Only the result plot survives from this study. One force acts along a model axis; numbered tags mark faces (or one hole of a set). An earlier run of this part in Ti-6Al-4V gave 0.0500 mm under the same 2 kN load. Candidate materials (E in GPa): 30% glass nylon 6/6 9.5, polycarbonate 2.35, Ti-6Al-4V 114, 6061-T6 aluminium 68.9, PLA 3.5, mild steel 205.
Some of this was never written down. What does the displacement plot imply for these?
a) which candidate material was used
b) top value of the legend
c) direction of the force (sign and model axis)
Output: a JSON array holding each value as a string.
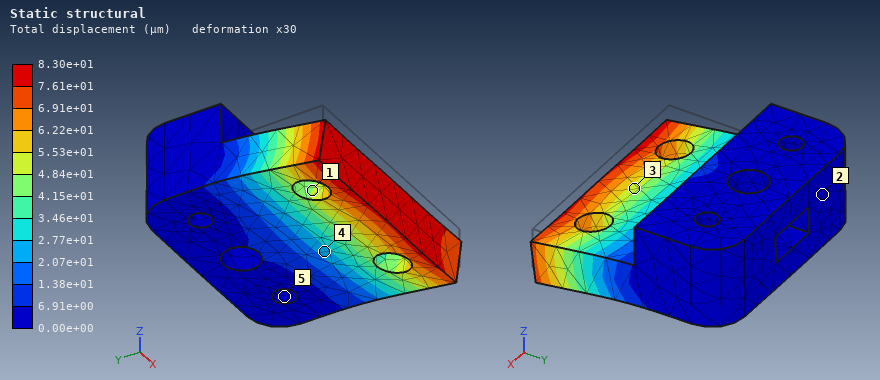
["6061-T6 aluminium", "8.30e+01 µm", "-Z"]
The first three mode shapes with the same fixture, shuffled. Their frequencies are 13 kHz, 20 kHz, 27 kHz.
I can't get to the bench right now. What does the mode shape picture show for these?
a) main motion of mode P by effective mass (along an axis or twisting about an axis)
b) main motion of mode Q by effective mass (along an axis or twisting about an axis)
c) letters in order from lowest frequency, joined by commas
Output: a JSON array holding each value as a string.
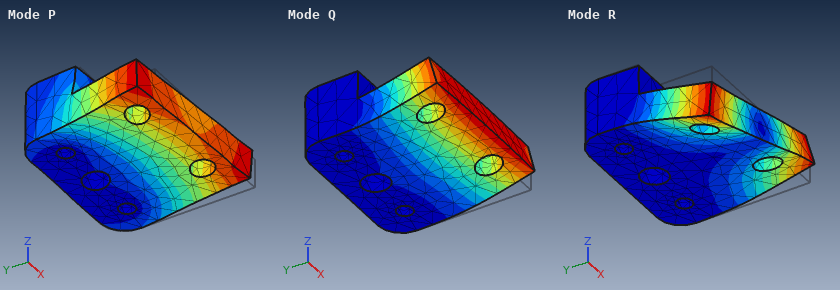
["along X", "along Z", "Q, R, P"]
